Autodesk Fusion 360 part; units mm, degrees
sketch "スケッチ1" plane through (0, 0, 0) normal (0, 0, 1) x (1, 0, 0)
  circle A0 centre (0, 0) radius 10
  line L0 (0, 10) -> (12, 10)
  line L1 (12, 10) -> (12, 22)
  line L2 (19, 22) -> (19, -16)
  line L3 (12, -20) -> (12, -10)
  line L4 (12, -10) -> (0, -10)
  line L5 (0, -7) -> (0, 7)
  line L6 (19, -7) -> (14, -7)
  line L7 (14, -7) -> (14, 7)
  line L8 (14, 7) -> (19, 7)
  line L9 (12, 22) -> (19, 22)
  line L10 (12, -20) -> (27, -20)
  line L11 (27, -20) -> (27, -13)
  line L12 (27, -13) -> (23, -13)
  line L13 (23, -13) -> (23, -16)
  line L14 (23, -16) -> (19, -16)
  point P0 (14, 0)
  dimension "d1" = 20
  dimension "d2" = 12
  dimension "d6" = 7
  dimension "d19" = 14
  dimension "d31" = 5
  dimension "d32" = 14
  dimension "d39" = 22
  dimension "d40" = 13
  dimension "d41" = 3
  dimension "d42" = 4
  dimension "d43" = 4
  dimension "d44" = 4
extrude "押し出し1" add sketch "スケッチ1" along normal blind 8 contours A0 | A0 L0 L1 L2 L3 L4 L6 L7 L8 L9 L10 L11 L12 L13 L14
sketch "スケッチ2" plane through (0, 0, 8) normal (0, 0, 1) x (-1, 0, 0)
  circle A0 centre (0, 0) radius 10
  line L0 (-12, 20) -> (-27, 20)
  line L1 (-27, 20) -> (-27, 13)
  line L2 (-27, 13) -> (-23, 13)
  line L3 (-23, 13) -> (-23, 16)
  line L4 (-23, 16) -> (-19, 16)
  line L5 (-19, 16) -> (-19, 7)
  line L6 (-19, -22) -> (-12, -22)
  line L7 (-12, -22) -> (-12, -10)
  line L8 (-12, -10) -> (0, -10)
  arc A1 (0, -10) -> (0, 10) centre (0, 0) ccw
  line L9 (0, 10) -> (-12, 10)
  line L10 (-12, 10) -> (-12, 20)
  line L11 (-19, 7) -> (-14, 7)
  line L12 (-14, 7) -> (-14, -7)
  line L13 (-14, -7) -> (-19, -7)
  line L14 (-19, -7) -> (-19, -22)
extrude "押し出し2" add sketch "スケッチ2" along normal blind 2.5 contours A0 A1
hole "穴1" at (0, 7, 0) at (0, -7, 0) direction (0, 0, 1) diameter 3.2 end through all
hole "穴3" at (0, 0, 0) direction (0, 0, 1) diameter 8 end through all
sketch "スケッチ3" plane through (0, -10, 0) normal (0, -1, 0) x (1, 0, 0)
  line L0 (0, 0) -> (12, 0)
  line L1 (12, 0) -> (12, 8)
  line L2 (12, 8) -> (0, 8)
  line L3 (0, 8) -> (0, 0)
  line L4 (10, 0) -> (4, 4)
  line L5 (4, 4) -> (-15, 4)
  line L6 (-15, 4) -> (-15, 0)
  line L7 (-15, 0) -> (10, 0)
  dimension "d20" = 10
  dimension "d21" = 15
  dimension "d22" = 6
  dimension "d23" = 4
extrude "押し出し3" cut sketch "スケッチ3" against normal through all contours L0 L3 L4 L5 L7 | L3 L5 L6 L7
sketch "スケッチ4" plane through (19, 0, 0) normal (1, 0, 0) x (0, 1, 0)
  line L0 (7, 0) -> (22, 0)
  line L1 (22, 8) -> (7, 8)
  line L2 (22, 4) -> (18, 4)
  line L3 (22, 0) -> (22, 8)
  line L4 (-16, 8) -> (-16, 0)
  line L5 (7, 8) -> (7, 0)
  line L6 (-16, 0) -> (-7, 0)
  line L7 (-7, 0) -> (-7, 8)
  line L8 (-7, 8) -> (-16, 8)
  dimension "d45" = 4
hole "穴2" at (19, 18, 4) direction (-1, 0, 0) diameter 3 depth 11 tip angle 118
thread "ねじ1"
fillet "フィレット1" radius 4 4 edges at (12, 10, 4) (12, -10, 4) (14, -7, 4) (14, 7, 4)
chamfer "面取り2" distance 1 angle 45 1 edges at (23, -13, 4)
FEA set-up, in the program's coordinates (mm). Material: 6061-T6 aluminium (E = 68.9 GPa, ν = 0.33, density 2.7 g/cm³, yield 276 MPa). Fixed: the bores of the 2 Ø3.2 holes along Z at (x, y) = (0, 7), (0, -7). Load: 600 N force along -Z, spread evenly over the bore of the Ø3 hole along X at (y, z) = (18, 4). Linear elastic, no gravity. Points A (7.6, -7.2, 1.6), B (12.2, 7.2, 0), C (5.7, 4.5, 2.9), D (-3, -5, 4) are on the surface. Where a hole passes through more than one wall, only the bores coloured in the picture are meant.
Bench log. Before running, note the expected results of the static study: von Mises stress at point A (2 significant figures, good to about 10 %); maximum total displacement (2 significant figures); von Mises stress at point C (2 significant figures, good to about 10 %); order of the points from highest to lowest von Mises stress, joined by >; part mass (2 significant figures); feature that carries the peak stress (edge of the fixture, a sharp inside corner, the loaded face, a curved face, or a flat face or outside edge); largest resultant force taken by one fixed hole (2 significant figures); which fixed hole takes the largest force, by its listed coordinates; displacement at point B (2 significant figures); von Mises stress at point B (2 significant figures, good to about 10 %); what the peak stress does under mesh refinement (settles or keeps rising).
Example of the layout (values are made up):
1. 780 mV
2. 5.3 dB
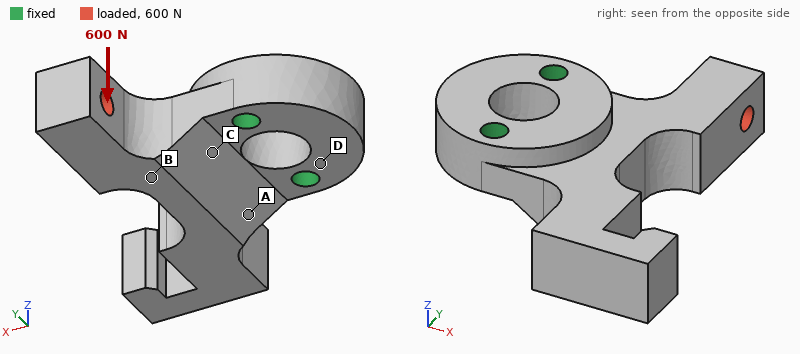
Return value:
1. 35 MPa
2. 0.16 mm
3. 75 MPa
4. B > C > A > D
5. 12 g
6. edge of the fixture
7. 930 N
8. (0, 7)
9. 0.053 mm
10. 91 MPa
11. keeps rising
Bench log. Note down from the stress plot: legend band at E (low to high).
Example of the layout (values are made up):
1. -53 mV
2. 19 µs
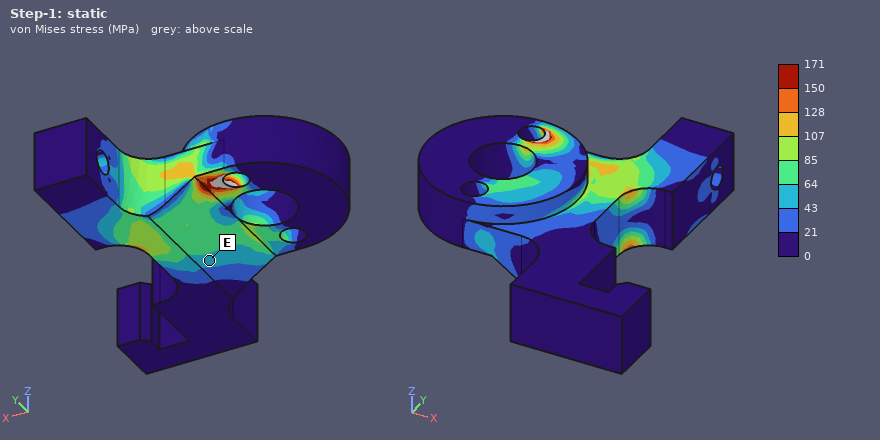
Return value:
1. 43 to 64 MPa
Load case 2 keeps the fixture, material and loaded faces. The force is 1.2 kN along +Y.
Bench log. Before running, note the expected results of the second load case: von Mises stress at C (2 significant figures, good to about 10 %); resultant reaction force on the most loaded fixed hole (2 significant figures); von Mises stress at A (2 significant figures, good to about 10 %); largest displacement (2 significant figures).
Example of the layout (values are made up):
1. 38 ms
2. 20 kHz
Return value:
1. 17 MPa
2. 1.4 kN
3. 14 MPa
4. 51 µm
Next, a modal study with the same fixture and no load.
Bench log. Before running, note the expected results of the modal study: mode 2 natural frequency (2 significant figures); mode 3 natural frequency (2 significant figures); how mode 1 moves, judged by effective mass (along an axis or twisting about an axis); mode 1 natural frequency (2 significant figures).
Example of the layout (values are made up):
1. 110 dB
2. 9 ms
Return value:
1. 8600 Hz
2. 9900 Hz
3. along Z
4. 6100 Hz
